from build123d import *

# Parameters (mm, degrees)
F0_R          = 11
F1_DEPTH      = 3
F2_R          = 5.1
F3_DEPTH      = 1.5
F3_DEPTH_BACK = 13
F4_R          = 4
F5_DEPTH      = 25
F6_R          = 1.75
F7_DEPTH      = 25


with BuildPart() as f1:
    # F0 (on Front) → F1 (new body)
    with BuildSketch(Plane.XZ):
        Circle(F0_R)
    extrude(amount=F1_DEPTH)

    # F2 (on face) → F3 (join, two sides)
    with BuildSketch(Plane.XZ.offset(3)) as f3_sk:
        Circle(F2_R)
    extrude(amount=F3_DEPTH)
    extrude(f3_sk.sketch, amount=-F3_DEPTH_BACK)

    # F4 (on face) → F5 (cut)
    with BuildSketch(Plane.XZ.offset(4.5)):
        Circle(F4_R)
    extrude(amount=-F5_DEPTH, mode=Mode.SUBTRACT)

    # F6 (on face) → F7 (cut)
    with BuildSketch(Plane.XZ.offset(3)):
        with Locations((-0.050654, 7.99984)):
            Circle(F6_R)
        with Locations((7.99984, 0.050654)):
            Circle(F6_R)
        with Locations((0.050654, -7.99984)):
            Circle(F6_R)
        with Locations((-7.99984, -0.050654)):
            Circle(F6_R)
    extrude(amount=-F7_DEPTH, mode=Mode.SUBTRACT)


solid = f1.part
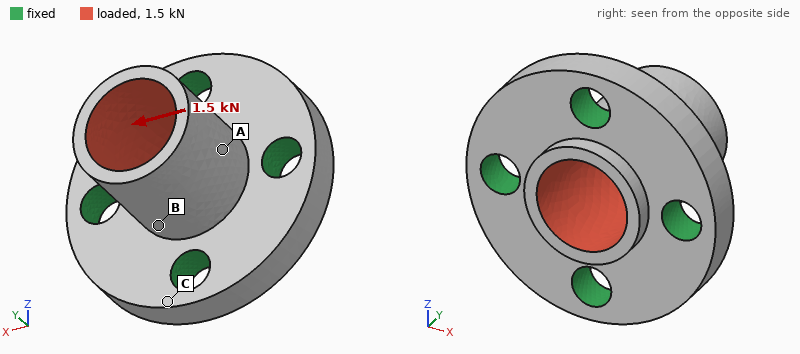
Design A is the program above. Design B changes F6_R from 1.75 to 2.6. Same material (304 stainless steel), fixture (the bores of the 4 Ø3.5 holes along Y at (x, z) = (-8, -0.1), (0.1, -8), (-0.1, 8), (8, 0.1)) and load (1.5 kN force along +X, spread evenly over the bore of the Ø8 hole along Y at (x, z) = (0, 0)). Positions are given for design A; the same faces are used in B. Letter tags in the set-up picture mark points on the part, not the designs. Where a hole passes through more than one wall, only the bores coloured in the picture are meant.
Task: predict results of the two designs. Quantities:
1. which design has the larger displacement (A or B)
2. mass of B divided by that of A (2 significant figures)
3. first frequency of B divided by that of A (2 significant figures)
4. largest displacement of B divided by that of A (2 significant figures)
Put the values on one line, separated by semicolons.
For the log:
A; 0.89; 1.1; 0.85
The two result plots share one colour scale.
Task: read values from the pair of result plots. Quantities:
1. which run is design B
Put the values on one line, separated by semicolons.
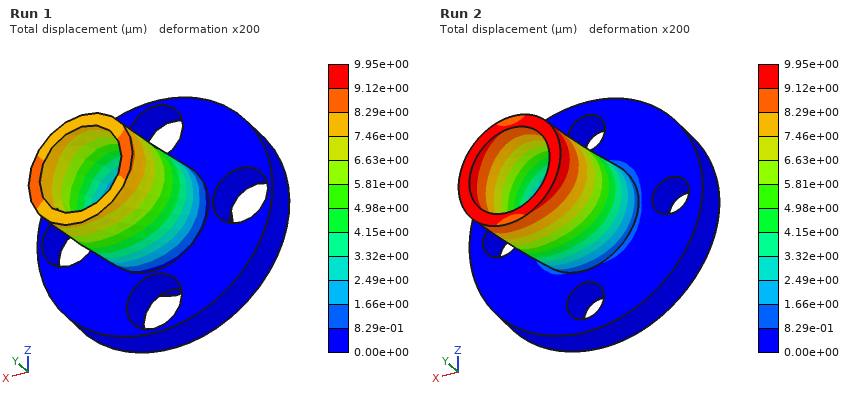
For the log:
Run 1
